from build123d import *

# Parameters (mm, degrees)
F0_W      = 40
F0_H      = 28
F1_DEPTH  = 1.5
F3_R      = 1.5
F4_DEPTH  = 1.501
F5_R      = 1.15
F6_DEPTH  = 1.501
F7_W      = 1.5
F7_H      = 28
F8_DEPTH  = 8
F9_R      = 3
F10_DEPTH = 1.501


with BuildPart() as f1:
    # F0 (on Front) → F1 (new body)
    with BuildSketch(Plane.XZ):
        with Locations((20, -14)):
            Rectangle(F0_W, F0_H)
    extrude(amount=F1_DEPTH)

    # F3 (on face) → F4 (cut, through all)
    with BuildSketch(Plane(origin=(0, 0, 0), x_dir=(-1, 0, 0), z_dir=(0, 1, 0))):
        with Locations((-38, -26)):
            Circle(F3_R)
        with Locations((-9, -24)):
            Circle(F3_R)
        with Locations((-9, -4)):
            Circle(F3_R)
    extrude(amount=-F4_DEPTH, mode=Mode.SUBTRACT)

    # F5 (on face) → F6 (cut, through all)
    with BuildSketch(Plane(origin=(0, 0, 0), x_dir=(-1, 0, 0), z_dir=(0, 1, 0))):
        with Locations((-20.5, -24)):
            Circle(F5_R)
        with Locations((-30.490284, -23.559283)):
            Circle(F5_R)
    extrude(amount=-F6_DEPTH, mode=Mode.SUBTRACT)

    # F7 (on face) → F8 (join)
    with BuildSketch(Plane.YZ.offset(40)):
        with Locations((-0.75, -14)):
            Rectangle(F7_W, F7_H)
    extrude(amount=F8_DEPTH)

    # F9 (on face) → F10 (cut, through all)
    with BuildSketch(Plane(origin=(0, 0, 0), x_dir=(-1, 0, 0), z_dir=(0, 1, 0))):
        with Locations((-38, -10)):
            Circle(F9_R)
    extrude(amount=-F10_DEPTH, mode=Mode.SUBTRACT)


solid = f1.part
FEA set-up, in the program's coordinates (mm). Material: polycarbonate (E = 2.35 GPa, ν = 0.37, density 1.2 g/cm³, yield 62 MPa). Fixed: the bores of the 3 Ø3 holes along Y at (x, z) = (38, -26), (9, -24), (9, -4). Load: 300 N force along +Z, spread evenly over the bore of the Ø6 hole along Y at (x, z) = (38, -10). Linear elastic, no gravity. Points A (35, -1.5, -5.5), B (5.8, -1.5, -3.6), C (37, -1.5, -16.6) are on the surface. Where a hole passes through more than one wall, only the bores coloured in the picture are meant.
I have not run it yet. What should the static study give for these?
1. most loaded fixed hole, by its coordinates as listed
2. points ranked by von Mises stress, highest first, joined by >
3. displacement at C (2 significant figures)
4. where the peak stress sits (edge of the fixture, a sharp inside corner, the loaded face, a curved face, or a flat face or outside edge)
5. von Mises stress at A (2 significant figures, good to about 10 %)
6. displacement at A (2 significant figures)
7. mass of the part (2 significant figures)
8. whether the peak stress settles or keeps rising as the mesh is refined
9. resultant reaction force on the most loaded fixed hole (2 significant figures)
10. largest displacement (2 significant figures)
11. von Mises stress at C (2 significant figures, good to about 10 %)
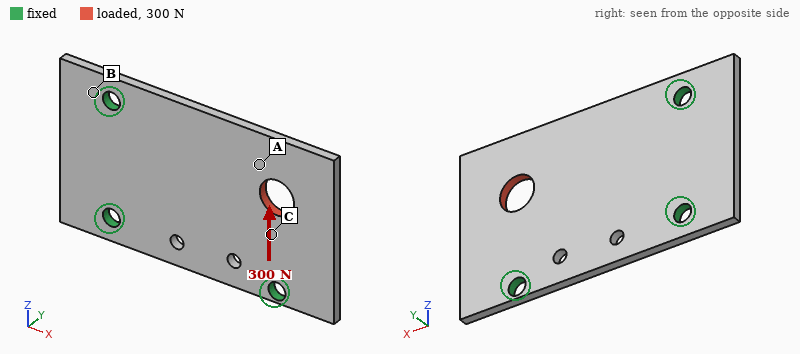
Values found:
(38, -26)
C > A > B
0.066 mm
edge of the fixture
9.8 MPa
0.12 mm
2.3 g
keeps rising
250 N
0.15 mm
15 MPa
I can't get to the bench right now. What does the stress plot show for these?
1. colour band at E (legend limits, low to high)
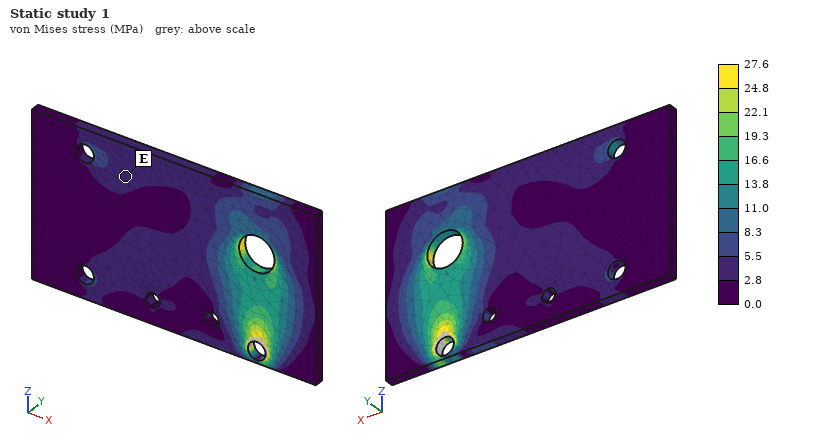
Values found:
2.8 to 5.5 MPa
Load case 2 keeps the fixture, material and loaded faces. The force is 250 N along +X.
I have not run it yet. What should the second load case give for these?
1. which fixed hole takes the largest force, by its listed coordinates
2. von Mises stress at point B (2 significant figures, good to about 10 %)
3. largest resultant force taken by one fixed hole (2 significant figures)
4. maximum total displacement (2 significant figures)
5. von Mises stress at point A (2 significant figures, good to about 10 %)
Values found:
(9, -4)
2.5 MPa
120 N
0.13 mm
11 MPa
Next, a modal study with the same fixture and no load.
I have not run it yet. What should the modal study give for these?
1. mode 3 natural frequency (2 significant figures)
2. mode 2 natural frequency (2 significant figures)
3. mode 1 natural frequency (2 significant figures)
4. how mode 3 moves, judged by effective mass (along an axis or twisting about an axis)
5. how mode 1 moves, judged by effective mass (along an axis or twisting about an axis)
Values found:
2700 Hz
1700 Hz
700 Hz
along Y
along Y
